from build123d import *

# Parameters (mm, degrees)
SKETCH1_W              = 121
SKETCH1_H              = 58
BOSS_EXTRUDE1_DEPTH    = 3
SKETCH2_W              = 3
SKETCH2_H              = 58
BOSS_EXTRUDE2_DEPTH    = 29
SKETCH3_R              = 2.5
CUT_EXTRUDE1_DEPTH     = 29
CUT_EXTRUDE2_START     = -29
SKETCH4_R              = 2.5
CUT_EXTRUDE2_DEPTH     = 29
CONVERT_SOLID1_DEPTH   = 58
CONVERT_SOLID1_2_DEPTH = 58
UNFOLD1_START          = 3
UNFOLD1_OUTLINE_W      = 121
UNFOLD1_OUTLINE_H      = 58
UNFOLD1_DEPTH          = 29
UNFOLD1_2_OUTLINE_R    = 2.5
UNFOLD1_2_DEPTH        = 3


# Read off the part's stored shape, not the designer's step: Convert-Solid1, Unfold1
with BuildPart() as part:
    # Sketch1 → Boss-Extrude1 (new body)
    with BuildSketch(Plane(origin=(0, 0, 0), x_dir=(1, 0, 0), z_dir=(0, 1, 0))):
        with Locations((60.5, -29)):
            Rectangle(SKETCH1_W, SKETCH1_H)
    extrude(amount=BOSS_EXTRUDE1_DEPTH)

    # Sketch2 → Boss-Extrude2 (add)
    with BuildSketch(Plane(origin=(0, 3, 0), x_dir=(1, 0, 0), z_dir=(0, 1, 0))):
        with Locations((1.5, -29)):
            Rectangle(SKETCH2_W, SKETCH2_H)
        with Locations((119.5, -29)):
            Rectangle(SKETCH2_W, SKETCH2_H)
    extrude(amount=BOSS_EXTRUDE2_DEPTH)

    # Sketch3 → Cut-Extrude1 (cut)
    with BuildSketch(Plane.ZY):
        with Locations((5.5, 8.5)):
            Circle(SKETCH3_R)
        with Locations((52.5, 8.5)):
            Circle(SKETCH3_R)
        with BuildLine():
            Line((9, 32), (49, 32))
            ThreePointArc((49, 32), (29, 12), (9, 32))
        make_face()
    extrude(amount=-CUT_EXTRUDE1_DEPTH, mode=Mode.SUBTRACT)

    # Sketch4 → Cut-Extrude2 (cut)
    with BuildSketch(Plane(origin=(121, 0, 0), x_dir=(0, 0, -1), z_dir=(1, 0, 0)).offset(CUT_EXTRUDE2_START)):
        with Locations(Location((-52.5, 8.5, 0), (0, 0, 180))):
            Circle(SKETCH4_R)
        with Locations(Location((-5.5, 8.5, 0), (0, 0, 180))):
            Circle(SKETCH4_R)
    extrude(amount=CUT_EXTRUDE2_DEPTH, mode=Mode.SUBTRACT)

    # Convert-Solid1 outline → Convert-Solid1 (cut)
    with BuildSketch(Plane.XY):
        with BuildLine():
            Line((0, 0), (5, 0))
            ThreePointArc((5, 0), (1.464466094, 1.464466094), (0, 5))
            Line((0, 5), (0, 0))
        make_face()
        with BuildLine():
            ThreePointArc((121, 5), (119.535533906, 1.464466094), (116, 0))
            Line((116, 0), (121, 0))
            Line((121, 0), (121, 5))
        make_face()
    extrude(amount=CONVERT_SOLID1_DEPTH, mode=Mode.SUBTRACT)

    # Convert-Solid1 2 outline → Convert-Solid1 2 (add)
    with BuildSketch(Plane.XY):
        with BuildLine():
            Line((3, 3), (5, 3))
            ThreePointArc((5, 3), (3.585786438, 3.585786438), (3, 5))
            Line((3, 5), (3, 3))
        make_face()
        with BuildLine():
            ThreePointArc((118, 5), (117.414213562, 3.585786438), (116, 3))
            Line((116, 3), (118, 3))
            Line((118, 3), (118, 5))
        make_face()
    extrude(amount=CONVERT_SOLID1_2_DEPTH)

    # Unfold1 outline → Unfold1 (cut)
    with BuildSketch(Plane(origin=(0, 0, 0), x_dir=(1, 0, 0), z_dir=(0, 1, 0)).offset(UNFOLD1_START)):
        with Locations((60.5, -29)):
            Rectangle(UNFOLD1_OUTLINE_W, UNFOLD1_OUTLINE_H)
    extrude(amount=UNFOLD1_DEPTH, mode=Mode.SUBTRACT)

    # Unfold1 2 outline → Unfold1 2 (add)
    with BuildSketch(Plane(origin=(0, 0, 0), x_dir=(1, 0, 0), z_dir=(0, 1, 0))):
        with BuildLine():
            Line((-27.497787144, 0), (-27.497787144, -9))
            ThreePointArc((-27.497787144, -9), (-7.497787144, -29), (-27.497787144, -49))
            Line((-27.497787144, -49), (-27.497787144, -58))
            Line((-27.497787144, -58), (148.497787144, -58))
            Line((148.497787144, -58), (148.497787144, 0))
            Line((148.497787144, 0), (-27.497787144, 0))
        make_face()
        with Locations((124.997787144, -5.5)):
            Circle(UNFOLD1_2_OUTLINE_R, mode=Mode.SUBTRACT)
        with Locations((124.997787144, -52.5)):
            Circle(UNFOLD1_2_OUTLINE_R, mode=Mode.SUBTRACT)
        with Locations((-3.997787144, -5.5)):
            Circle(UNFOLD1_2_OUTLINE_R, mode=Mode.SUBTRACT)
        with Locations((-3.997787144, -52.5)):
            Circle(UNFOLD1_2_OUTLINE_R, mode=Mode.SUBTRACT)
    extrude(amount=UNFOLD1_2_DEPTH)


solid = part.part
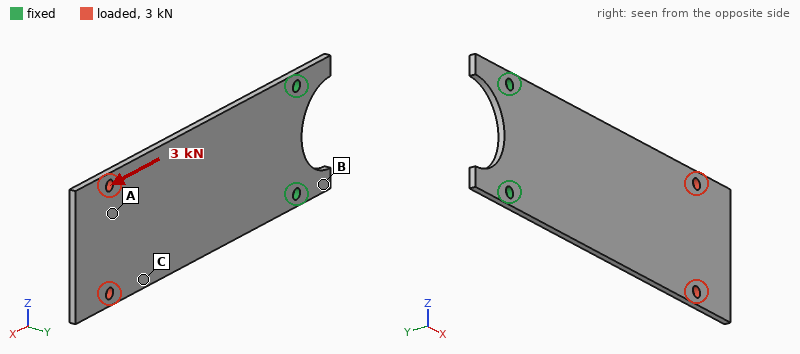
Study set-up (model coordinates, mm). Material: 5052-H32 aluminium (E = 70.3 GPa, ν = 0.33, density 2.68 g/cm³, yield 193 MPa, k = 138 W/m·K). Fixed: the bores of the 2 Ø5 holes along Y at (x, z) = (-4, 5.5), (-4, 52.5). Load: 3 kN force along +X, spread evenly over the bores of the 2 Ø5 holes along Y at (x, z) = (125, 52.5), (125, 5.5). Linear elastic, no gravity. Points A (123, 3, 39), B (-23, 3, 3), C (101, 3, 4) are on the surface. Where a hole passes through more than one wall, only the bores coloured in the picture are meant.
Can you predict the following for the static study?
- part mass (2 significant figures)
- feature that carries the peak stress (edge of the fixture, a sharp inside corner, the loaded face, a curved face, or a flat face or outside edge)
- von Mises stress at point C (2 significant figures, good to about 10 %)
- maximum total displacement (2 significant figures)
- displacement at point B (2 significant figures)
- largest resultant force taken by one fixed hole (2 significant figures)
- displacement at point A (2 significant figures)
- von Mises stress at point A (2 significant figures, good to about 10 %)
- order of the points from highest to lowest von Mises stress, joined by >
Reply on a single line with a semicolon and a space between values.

76 g; edge of the fixture; 20 MPa; 40 µm; 7.6 µm; 1.6 kN; 33 µm; 11 MPa; C > A > B
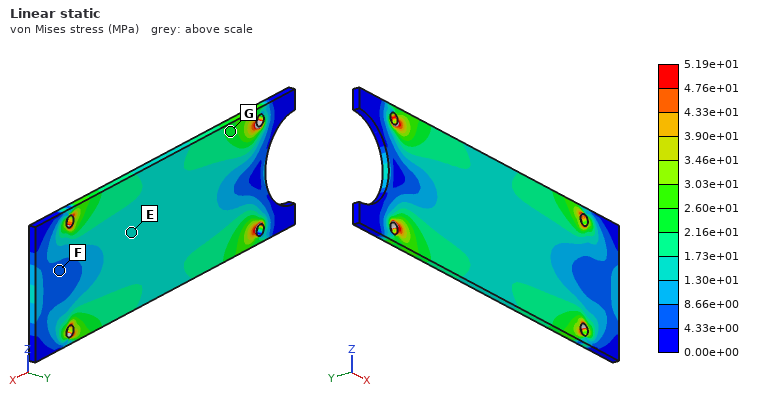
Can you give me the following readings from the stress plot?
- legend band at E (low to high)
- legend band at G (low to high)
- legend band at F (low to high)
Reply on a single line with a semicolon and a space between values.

1.30e+01 to 1.73e+01 MPa; 2.16e+01 to 2.60e+01 MPa; 4.33e+00 to 8.66e+00 MPa
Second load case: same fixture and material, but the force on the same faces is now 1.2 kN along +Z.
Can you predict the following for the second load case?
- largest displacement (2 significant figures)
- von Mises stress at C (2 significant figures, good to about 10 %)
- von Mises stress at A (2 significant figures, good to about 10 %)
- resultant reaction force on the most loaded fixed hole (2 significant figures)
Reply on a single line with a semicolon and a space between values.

0.38 mm; 15 MPa; 12 MPa; 3.3 kN
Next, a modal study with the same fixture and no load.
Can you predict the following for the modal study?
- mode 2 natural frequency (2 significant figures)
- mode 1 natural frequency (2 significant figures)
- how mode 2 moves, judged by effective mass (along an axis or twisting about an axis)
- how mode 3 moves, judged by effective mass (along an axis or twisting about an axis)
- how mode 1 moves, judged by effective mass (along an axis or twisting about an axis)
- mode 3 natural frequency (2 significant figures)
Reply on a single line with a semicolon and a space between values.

590 Hz; 100 Hz; twisting about X; along Y; along Y; 660 Hz
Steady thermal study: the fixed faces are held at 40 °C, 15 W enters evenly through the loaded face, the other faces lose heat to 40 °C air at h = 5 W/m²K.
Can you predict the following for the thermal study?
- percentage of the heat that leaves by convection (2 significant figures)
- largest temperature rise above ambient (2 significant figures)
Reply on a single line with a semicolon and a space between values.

25 %; 74 K
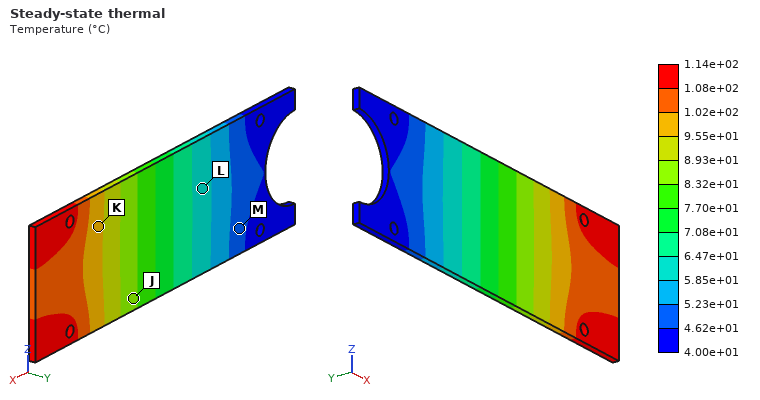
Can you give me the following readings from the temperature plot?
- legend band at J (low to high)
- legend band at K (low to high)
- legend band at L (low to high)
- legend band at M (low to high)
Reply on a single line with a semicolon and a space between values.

8.32e+01 to 8.93e+01 °C; 9.55e+01 to 1.02e+02 °C; 5.85e+01 to 6.47e+01 °C; 4.62e+01 to 5.23e+01 °C
